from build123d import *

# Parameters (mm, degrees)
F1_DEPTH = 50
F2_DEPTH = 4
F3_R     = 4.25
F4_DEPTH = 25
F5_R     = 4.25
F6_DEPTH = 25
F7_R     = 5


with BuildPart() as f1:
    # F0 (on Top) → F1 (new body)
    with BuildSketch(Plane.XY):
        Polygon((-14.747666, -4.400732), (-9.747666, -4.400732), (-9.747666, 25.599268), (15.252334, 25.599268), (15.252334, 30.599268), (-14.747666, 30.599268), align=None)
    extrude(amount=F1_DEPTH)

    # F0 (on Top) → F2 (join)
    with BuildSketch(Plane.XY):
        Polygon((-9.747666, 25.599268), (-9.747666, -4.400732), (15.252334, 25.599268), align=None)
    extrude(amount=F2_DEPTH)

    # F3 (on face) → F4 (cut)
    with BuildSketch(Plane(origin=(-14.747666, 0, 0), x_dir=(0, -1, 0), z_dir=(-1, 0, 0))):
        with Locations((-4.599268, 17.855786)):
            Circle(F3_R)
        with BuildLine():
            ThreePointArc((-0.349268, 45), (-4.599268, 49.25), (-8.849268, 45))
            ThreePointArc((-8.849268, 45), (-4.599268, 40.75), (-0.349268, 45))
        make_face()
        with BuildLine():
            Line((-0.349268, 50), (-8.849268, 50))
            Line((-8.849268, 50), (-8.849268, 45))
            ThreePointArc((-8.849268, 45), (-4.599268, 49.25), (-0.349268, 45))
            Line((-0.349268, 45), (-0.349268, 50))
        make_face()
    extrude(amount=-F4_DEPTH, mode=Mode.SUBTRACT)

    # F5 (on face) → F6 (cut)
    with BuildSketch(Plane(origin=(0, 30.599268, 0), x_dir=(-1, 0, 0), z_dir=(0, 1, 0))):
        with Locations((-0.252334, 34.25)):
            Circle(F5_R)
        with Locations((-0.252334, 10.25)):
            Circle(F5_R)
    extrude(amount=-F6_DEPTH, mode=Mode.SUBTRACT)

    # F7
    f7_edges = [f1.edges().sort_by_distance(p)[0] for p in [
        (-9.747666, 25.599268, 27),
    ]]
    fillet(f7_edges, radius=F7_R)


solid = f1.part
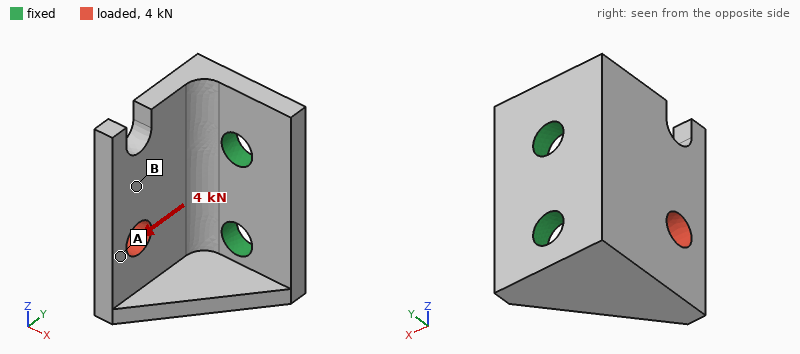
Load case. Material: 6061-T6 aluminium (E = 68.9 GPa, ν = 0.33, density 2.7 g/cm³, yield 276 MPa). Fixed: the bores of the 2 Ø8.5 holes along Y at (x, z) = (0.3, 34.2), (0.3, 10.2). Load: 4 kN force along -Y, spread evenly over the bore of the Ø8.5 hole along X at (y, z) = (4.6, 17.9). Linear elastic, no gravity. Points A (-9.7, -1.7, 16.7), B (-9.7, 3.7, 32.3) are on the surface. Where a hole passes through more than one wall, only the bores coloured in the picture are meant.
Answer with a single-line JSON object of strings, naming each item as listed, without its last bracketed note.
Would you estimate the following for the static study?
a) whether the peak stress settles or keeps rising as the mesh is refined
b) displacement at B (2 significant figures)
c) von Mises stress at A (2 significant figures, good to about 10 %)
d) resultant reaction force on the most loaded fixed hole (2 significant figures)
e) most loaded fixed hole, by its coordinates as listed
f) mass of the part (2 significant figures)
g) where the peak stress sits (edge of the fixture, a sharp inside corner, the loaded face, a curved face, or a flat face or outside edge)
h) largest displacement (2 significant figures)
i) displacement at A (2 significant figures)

{"whether the peak stress settles or keeps rising as the mesh is refined": "keeps rising", "displacement at B": "0.094 mm", "von Mises stress at A": "45 MPa", "resultant reaction force on the most loaded fixed hole": "2.6 kN", "most loaded fixed hole, by its coordinates as listed": "(0.3, 10.2)", "mass of the part": "42 g", "where the peak stress sits": "edge of the fixture", "largest displacement": "0.13 mm", "displacement at A": "0.11 mm"}
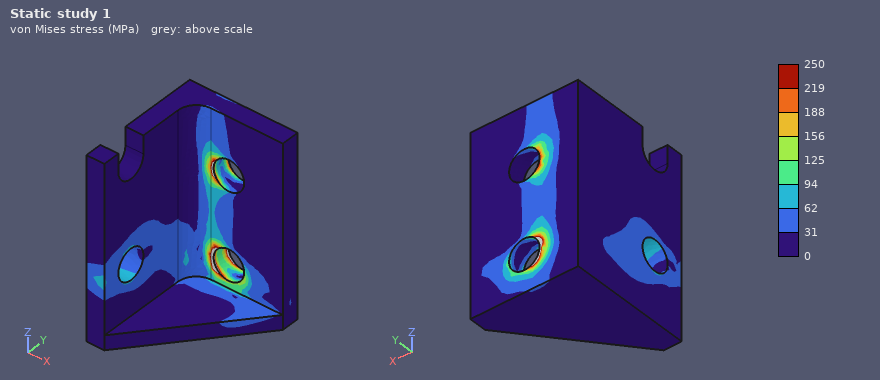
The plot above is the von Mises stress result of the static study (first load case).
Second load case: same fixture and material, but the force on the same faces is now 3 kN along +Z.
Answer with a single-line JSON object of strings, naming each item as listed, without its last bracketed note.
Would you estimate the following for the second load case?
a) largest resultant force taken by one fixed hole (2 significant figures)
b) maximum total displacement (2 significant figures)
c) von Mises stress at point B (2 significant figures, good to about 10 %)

{"largest resultant force taken by one fixed hole": "2.9 kN", "maximum total displacement": "0.13 mm", "von Mises stress at point B": "31 MPa"}
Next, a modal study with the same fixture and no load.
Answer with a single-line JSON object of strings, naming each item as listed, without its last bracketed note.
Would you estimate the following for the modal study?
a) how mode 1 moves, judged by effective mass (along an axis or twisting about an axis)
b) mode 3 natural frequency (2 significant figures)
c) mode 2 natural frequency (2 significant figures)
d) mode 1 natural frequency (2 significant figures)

{"how mode 1 moves, judged by effective mass": "along X", "mode 3 natural frequency": "9900 Hz", "mode 2 natural frequency": "6500 Hz", "mode 1 natural frequency": "4100 Hz"}
